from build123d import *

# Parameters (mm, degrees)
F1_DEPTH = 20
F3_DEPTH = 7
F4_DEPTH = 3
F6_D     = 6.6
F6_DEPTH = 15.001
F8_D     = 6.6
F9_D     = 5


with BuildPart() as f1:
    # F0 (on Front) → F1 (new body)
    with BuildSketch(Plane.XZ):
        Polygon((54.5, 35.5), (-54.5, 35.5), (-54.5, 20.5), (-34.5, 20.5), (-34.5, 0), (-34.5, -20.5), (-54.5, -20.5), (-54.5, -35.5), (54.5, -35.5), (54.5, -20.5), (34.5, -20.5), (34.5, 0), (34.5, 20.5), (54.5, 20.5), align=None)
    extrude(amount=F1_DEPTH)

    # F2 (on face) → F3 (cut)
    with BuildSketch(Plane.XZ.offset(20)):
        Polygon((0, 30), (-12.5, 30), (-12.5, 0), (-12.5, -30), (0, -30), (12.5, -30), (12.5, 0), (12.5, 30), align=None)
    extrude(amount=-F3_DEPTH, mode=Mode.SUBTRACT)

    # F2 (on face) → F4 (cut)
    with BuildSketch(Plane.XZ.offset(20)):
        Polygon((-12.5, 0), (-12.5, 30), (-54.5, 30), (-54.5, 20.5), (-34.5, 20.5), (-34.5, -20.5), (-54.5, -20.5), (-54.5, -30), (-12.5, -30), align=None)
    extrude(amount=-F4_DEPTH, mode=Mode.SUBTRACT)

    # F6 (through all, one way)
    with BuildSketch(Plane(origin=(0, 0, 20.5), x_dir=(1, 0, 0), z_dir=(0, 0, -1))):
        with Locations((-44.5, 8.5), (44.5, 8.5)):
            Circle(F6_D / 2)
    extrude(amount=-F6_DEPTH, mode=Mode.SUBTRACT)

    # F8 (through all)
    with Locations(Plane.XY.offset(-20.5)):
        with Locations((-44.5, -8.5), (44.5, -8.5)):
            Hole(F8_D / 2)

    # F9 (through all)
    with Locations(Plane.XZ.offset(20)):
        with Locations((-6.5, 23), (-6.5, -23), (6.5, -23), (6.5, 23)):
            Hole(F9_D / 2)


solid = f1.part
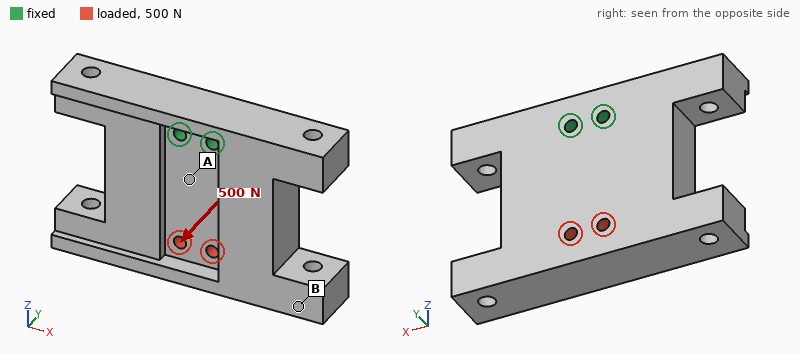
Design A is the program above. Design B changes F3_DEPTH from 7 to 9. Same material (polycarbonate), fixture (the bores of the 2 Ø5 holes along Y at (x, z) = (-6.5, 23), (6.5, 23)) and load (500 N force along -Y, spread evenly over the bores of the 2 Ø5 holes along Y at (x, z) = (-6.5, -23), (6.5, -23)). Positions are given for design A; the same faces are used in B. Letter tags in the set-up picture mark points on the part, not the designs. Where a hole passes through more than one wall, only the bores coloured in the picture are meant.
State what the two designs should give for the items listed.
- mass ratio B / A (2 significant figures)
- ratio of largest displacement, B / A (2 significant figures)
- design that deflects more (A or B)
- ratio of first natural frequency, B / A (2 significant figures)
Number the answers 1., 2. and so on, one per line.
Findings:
1. 0.97
2. 1.3
3. B
4. 0.87
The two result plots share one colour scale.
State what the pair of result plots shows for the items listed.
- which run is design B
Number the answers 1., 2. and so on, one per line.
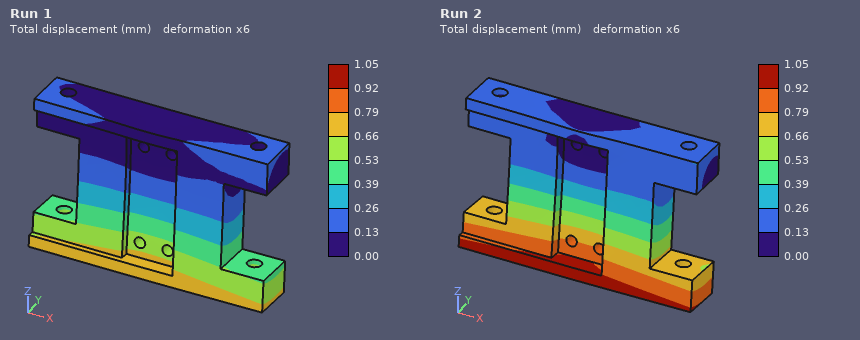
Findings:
1. Run 2
